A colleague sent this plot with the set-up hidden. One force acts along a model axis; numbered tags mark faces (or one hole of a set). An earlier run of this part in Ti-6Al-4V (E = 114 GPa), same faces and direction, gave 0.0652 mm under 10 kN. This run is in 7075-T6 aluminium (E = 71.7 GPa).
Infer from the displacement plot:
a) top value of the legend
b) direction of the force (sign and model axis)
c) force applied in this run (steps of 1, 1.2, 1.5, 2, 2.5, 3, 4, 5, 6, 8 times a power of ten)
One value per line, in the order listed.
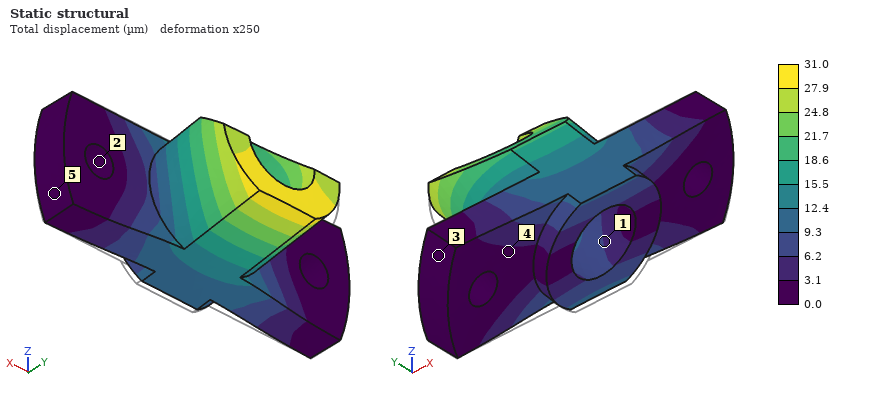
31.0 µm
+Z
3 kN
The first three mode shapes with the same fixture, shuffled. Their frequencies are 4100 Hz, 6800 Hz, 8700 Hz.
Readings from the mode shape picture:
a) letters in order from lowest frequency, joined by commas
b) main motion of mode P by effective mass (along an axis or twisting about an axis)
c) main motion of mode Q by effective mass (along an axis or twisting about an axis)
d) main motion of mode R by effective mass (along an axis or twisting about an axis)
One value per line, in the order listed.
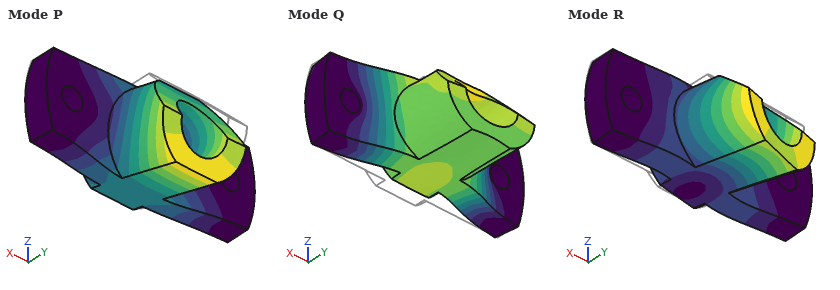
P, Q, R
along Z
along Y
along X
